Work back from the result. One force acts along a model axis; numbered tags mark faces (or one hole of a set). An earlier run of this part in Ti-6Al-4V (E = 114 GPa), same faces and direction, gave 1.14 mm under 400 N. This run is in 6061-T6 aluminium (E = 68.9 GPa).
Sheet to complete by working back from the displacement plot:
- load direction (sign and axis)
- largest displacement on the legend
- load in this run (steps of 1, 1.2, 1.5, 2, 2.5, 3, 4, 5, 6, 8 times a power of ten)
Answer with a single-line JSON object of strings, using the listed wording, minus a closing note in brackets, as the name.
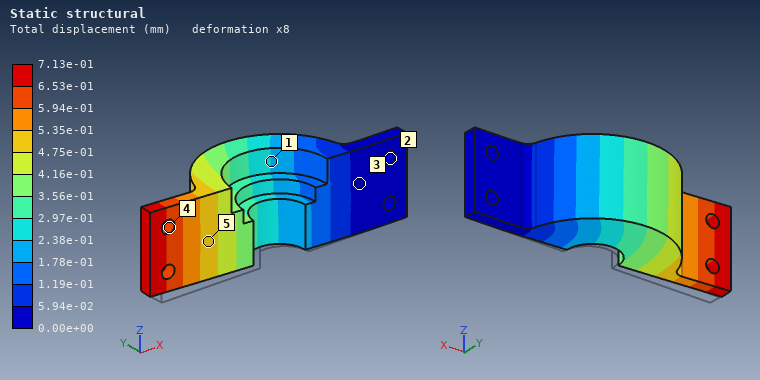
{"load direction": "+Y", "largest displacement on the legend": "7.13e-01 mm", "load in this run": "150 N"}
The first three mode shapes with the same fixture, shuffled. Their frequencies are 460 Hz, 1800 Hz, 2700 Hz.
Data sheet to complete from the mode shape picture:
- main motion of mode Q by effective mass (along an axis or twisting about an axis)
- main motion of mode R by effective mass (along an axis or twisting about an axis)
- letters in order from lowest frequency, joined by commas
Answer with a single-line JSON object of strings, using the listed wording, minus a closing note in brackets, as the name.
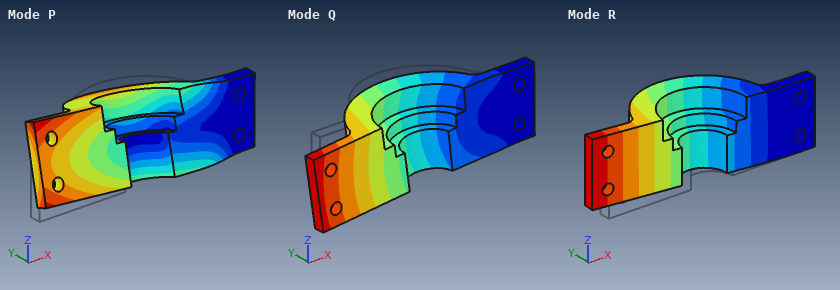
{"main motion of mode Q by effective mass": "along Z", "main motion of mode R by effective mass": "along Y", "letters in order from lowest frequency, joined by commas": "R, Q, P"}
